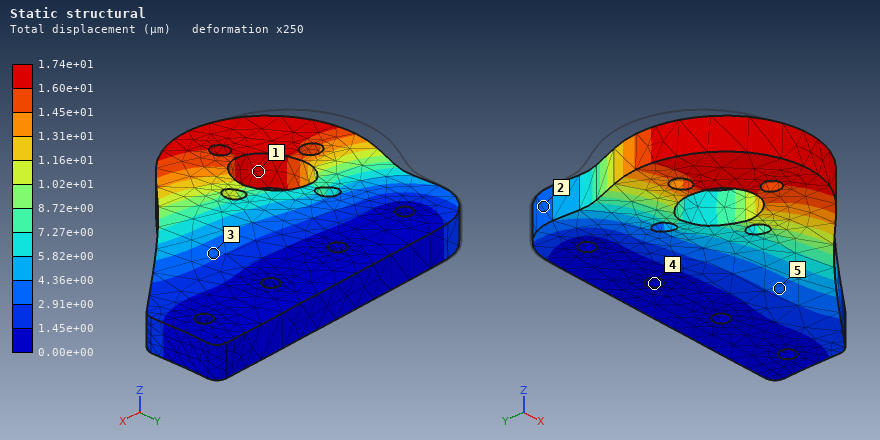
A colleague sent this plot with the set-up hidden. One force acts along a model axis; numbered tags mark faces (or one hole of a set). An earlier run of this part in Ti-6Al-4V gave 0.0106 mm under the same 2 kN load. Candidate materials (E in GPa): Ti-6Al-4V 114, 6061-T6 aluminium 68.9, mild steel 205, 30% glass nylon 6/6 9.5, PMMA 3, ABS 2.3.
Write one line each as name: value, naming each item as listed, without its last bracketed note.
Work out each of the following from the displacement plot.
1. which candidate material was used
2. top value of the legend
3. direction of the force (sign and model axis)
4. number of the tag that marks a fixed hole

which candidate material was used: 6061-T6 aluminium
top value of the legend: 1.74e+01 µm
direction of the force: +X
number of the tag that marks a fixed hole: 4
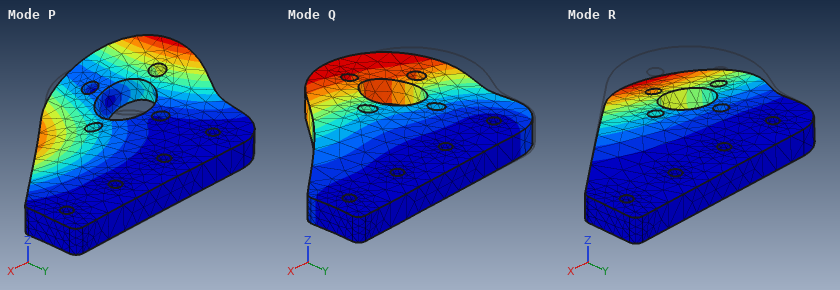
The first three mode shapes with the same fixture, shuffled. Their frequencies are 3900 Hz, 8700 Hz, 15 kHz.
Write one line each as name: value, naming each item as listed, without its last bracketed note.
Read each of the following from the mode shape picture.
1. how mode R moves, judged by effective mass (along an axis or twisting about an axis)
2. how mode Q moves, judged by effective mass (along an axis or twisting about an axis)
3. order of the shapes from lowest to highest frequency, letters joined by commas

how mode R moves, judged by effective mass: along Z
how mode Q moves, judged by effective mass: along X
order of the shapes from lowest to highest frequency, letters joined by commas: R, P, Q
